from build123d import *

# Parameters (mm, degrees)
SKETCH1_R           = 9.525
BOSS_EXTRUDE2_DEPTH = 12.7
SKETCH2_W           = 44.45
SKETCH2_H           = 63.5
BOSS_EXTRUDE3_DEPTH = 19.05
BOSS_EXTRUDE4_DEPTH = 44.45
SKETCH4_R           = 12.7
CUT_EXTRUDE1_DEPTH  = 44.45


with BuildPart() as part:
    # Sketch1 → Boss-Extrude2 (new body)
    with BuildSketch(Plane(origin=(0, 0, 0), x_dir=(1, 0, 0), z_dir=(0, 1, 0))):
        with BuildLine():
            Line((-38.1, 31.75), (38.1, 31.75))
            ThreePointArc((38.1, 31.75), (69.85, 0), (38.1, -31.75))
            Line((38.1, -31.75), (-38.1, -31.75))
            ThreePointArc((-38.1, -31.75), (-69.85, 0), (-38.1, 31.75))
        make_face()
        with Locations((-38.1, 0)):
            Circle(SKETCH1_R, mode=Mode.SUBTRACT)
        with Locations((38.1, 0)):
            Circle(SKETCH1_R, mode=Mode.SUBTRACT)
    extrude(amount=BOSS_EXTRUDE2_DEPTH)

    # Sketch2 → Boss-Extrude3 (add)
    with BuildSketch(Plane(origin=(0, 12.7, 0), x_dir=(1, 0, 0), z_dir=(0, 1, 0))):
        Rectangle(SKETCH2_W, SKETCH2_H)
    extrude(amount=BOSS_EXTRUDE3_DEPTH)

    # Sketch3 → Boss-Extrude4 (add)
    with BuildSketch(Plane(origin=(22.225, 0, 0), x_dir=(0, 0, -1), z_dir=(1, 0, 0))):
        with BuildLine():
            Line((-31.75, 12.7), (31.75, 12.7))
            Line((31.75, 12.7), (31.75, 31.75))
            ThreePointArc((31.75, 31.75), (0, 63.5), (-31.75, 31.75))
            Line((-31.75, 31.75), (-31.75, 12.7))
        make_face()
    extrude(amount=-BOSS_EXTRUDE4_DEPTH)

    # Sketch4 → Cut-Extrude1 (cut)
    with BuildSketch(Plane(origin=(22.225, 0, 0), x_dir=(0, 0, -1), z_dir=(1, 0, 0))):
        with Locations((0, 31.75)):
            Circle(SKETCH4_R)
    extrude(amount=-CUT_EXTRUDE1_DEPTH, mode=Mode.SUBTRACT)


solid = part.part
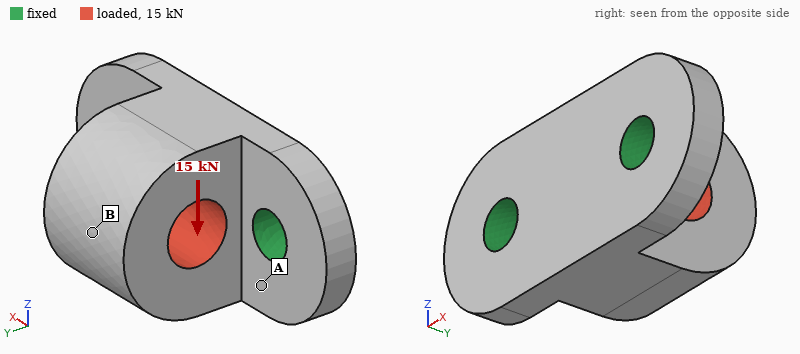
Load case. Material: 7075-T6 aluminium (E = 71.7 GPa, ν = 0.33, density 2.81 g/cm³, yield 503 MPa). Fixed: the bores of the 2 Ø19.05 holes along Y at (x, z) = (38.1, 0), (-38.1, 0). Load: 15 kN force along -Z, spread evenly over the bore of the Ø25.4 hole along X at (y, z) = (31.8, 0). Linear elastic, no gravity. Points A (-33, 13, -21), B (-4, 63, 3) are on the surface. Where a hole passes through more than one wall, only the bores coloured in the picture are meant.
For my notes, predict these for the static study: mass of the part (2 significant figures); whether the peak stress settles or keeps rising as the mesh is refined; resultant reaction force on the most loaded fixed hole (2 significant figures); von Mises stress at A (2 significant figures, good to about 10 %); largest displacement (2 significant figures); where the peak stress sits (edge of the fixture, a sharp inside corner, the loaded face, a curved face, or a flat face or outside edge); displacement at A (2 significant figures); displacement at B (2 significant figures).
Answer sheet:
550 g
keeps rising
7.5 kN
37 MPa
0.13 mm
edge of the fixture
0.022 mm
0.13 mm
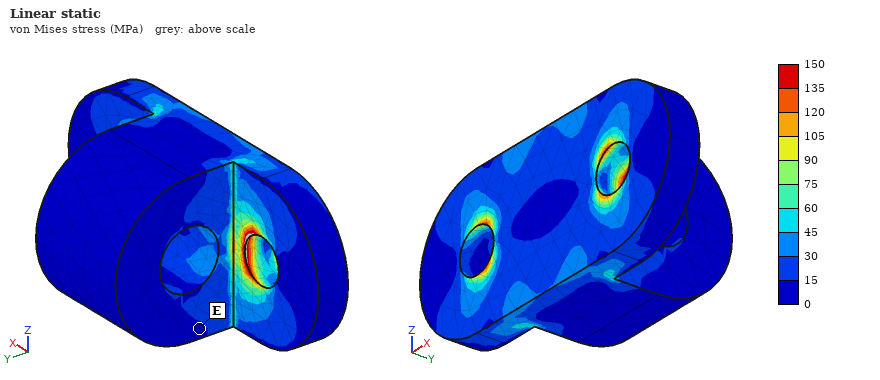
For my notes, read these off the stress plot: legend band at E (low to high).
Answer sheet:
0 to 15 MPa
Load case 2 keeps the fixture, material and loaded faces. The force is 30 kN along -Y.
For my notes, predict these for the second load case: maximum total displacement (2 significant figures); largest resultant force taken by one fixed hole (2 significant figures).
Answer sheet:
43 µm
16 kN
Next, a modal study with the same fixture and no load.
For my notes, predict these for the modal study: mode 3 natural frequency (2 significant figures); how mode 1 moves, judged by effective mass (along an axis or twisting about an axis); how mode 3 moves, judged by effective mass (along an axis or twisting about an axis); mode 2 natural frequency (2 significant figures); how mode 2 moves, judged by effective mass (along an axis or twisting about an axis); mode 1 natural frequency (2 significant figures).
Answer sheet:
7400 Hz
along Z
along Y
5800 Hz
along X
3200 Hz
